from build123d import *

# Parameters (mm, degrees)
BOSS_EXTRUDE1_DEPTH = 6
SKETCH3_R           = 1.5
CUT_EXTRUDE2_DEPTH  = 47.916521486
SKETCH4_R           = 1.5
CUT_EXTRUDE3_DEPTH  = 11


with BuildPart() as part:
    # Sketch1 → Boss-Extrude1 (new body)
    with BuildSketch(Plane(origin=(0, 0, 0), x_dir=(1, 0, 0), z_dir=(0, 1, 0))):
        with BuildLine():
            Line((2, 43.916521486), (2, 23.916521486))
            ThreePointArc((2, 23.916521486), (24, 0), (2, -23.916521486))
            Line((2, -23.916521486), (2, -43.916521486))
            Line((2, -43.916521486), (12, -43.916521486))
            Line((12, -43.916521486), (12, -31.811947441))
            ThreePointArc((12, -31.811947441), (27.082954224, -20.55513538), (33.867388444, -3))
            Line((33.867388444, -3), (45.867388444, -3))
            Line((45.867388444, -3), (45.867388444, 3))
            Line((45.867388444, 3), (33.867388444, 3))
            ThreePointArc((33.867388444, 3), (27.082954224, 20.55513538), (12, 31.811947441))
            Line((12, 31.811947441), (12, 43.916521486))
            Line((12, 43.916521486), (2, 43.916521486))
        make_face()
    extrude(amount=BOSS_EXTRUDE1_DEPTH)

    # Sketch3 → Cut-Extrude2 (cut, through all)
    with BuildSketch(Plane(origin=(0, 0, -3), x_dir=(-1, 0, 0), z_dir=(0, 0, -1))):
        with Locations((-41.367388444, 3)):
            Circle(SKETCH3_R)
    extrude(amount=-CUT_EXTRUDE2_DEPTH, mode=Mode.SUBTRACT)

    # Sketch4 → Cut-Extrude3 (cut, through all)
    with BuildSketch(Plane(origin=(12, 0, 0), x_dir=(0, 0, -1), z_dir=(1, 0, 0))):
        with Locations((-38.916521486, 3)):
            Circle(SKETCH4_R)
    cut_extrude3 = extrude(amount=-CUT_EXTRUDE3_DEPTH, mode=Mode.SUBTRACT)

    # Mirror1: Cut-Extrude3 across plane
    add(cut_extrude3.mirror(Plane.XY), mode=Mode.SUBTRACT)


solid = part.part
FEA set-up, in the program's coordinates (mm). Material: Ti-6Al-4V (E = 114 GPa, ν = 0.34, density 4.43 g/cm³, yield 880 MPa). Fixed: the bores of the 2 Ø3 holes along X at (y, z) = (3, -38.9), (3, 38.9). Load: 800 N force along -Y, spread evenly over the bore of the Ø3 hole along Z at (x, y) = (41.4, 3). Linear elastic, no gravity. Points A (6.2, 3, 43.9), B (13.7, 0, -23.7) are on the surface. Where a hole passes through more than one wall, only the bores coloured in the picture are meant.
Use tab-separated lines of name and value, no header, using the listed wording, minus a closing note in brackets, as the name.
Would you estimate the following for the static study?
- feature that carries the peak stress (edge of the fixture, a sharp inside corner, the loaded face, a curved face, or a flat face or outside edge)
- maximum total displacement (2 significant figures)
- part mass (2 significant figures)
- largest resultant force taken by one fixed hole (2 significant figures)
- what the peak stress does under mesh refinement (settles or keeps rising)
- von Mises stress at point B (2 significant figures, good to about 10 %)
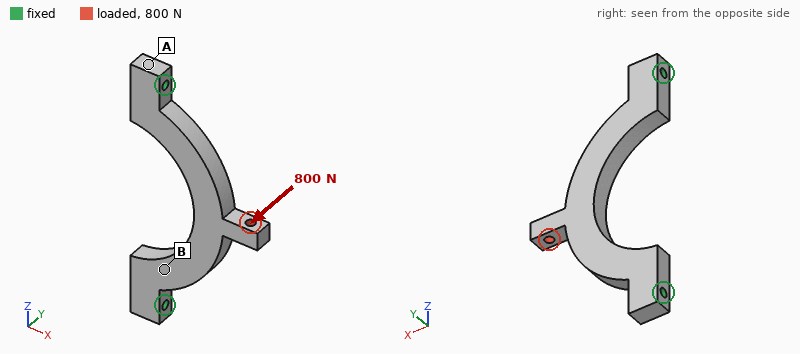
feature that carries the peak stress	edge of the fixture
maximum total displacement	0.78 mm
part mass	30 g
largest resultant force taken by one fixed hole	400 N
what the peak stress does under mesh refinement	keeps rising
von Mises stress at point B	180 MPa
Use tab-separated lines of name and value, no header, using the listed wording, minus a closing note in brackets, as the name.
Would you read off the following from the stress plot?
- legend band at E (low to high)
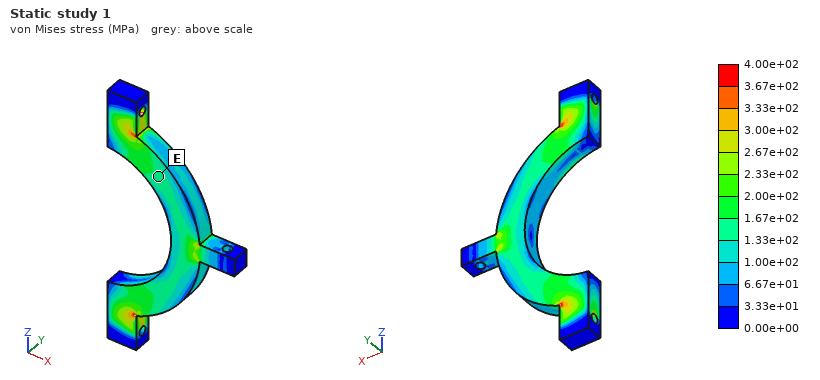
legend band at E	1.33e+02 to 1.67e+02 MPa
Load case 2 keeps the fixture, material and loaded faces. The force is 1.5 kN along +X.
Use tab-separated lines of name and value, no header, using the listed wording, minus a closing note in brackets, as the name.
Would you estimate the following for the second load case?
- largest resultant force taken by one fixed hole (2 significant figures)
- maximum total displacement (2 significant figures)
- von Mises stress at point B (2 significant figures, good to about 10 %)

largest resultant force taken by one fixed hole	1.1 kN
maximum total displacement	22 µm
von Mises stress at point B	23 MPa
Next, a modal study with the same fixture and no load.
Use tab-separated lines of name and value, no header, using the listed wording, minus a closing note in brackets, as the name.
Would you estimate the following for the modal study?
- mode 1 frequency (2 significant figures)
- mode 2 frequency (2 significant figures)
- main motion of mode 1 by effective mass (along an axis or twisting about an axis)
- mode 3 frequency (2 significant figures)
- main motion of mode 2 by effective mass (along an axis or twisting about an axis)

mode 1 frequency	2500 Hz
mode 2 frequency	8400 Hz
main motion of mode 1 by effective mass	along Y
mode 3 frequency	9800 Hz
main motion of mode 2 by effective mass	twisting about X
